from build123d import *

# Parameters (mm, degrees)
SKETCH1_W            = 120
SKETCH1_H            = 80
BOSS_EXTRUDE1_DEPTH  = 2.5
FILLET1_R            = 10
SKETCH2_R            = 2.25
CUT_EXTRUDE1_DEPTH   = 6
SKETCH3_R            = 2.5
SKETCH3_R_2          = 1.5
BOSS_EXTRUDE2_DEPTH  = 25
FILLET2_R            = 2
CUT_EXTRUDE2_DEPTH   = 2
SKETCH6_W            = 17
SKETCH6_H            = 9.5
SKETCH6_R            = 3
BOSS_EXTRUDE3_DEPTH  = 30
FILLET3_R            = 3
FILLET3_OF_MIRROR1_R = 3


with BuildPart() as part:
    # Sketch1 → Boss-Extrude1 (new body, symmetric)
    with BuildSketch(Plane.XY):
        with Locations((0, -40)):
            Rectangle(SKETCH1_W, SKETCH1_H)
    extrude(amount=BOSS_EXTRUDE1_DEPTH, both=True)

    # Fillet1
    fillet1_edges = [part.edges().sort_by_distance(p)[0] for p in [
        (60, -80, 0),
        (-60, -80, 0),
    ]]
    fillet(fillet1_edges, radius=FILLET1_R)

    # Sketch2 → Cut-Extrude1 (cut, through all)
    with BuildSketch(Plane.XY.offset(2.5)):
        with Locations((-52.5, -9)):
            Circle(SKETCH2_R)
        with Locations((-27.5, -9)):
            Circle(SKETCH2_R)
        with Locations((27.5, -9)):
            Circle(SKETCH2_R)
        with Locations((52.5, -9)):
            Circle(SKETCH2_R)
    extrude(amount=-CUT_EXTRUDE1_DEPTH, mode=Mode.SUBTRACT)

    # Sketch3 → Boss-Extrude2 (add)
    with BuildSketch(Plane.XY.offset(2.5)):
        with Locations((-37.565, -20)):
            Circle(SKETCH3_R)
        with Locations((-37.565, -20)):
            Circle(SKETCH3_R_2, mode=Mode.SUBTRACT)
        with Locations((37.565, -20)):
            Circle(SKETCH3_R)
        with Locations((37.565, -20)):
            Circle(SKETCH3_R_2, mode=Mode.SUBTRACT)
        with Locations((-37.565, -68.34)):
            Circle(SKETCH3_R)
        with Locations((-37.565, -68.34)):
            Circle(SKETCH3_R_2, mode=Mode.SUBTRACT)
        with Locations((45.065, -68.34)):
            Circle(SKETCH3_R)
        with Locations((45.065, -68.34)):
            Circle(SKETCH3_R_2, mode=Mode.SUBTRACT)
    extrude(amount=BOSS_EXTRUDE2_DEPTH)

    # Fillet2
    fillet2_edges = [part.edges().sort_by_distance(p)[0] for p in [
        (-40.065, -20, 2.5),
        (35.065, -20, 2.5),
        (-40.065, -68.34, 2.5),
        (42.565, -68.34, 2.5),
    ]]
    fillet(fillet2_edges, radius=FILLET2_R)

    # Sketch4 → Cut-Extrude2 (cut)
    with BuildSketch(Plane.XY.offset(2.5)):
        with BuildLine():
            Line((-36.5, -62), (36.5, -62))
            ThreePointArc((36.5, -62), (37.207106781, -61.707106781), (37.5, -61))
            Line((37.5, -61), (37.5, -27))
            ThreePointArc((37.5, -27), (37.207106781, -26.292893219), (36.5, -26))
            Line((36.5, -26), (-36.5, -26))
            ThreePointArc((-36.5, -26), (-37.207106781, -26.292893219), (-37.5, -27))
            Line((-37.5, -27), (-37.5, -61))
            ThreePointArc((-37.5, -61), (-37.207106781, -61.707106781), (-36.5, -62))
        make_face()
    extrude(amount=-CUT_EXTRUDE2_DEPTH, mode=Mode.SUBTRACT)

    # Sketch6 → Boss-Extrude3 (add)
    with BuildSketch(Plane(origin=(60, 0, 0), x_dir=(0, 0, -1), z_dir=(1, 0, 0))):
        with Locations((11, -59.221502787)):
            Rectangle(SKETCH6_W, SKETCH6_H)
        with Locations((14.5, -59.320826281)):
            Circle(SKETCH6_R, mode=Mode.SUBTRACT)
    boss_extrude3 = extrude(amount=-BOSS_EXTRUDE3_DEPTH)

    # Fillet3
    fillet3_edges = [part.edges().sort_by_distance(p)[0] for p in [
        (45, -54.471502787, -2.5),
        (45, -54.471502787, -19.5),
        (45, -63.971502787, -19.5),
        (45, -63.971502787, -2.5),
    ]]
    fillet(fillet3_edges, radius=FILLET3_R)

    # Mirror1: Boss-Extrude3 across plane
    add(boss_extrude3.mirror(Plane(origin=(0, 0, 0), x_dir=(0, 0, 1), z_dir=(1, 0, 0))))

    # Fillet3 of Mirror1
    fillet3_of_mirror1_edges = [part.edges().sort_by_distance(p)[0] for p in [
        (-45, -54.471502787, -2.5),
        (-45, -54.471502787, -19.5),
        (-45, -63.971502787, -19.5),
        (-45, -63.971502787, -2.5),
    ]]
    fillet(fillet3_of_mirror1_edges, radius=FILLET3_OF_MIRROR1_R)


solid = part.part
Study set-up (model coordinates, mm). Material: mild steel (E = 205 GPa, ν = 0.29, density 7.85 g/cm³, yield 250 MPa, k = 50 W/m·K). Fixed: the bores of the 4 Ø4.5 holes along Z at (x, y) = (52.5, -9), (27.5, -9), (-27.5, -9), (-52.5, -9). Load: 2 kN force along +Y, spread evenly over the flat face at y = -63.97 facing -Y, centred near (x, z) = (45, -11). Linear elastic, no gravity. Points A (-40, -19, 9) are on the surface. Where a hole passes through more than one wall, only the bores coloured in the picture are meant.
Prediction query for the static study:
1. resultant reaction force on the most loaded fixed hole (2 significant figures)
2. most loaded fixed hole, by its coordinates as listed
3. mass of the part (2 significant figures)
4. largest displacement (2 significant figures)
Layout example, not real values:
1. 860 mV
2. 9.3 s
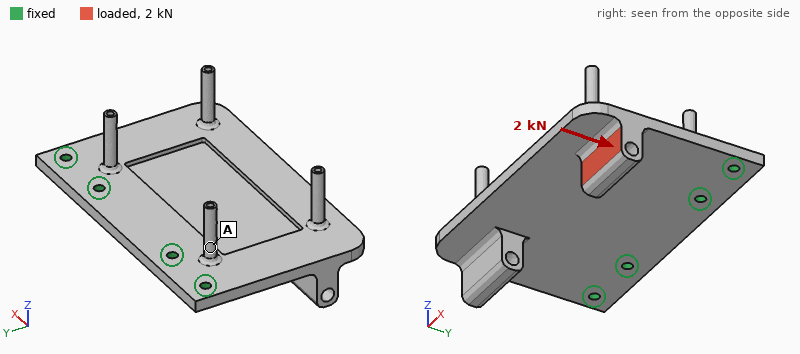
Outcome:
1. 1.3 kN
2. (27.5, -9)
3. 400 g
4. 0.41 mm
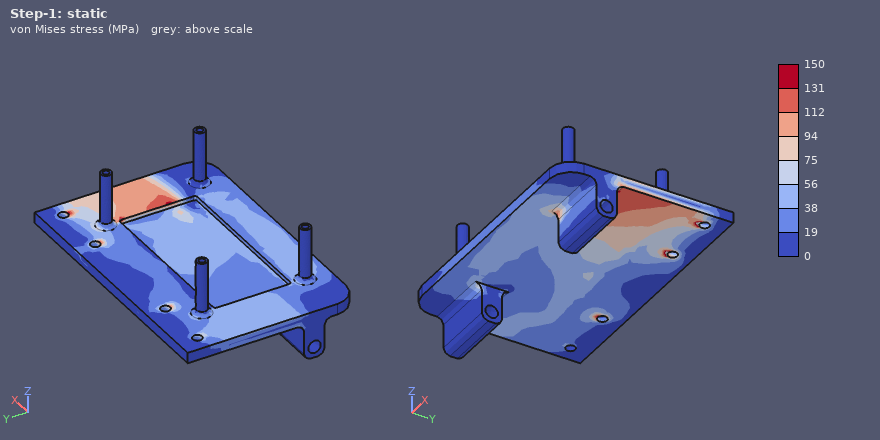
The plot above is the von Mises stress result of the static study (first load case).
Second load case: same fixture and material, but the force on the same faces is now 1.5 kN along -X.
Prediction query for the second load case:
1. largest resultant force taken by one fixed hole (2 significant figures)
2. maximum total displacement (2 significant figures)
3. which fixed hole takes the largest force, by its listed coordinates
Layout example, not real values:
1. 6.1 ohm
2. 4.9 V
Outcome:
1. 940 N
2. 0.10 mm
3. (52.5, -9)
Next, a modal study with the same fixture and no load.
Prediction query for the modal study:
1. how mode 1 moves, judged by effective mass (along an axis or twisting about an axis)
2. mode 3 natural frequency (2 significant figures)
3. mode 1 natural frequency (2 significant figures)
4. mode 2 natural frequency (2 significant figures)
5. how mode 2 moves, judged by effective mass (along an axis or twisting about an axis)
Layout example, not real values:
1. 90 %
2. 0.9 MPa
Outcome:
1. along Z
2. 2300 Hz
3. 610 Hz
4. 1000 Hz
5. twisting about Y
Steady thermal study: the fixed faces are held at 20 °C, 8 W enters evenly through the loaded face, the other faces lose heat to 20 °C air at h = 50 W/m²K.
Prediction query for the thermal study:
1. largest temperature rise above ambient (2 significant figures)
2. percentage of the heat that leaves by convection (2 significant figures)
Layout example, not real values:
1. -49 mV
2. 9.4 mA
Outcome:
1. 21 K
2. 69 %
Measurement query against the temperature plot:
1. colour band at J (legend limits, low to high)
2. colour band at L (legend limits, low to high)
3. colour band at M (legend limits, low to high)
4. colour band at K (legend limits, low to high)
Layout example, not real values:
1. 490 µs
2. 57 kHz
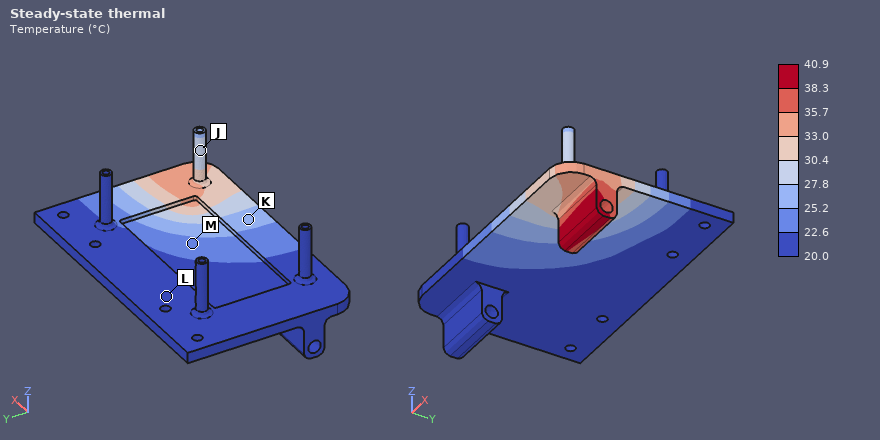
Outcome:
1. 27.8 to 30.4 °C
2. 20.0 to 22.6 °C
3. 22.6 to 25.2 °C
4. 25.2 to 27.8 °C
